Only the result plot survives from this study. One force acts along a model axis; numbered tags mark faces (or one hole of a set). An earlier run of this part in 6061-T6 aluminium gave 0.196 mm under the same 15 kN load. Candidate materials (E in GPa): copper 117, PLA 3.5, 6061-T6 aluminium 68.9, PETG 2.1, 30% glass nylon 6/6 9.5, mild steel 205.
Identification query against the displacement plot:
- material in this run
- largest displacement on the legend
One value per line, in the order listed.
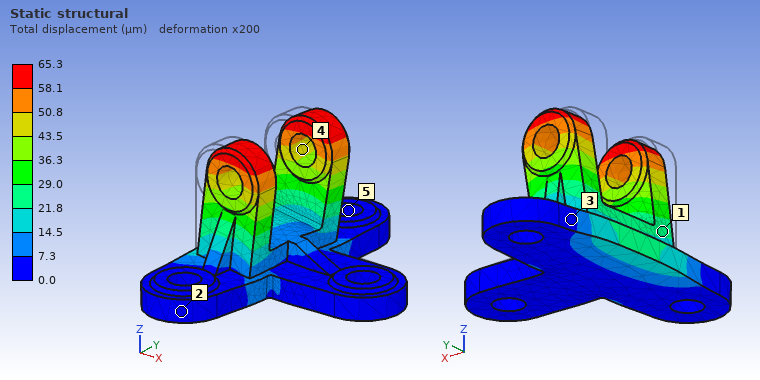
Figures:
mild steel
65.3 µm
